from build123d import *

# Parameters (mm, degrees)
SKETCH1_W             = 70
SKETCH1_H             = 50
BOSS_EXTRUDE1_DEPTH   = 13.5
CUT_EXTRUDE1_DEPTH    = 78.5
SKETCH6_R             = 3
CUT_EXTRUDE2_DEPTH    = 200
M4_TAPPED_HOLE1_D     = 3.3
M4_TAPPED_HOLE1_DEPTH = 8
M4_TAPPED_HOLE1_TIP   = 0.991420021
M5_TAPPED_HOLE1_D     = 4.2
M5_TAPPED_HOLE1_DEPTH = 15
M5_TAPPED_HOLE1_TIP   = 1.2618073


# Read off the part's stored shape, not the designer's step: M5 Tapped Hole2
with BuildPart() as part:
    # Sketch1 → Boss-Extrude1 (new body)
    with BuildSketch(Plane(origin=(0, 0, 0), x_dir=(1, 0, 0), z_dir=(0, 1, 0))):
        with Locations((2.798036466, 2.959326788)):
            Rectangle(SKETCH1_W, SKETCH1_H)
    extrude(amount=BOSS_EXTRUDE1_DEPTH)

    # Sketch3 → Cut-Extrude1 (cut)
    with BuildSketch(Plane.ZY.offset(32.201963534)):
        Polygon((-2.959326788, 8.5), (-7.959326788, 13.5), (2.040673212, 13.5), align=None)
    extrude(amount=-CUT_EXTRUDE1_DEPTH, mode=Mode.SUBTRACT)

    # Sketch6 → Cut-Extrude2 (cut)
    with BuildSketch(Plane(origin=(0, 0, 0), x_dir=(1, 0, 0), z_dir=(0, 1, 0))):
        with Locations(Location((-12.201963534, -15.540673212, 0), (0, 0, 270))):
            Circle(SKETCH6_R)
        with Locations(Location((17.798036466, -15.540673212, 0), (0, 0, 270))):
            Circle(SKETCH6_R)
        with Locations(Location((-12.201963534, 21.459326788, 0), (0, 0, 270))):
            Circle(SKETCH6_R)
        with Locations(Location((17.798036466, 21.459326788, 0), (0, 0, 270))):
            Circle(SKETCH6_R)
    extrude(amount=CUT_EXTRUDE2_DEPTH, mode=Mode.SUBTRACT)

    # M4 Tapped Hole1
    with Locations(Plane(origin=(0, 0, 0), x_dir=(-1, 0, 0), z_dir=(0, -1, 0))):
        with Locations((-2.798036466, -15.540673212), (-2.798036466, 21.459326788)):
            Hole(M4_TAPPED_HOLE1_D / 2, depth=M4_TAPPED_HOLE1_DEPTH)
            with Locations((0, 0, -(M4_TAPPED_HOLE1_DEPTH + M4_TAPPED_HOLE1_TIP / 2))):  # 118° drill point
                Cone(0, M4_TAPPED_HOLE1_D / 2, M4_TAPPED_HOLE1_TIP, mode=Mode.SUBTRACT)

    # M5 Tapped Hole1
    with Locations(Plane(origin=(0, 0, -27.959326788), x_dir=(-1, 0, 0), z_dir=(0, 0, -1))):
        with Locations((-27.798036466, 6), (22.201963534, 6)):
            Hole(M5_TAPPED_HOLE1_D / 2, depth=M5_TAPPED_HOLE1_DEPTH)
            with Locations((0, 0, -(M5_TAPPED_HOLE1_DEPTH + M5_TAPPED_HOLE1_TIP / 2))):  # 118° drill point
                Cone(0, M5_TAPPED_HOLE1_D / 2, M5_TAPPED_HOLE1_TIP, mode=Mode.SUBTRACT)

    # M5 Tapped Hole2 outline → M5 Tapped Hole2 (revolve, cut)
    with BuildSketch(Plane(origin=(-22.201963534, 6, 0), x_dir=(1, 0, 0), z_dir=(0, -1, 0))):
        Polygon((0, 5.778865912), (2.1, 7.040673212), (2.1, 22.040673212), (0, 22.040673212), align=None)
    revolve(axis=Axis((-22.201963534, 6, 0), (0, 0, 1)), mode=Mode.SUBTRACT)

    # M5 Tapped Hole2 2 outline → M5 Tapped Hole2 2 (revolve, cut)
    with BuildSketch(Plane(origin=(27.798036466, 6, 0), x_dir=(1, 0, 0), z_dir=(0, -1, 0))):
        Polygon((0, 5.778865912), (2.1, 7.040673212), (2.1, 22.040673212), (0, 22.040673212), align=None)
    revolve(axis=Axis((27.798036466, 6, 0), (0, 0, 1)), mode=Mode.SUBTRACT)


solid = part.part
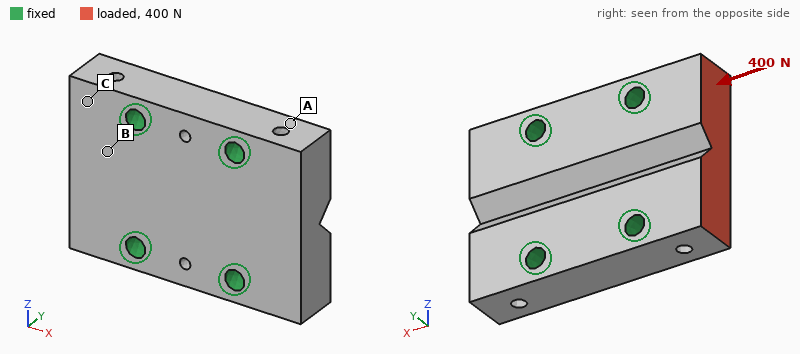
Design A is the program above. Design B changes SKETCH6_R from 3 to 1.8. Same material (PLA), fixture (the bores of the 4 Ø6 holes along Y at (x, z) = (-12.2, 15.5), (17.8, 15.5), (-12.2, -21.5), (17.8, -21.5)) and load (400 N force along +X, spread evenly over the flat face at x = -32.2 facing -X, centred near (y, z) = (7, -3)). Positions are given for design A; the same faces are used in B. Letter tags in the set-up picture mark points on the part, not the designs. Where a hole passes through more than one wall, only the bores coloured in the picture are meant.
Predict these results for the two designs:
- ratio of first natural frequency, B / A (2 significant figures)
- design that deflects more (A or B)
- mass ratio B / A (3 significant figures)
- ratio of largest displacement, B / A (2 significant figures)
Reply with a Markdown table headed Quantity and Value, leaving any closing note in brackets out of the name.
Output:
| Quantity | Value |
|---|---|
| ratio of first natural frequency, B / A | 0.87 |
| design that deflects more | B |
| mass ratio B / A | 1.02 |
| ratio of largest displacement, B / A | 1.1 |
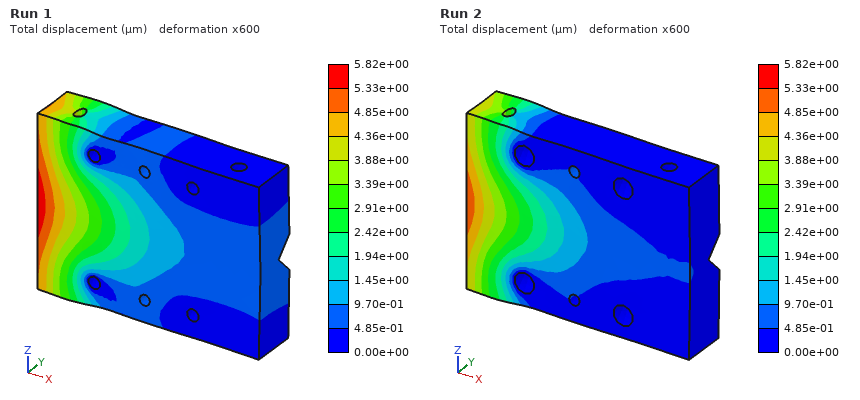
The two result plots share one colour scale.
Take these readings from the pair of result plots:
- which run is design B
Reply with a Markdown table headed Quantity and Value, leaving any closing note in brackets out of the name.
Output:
| Quantity | Value |
|---|---|
| which run is design B | Run 1 |
